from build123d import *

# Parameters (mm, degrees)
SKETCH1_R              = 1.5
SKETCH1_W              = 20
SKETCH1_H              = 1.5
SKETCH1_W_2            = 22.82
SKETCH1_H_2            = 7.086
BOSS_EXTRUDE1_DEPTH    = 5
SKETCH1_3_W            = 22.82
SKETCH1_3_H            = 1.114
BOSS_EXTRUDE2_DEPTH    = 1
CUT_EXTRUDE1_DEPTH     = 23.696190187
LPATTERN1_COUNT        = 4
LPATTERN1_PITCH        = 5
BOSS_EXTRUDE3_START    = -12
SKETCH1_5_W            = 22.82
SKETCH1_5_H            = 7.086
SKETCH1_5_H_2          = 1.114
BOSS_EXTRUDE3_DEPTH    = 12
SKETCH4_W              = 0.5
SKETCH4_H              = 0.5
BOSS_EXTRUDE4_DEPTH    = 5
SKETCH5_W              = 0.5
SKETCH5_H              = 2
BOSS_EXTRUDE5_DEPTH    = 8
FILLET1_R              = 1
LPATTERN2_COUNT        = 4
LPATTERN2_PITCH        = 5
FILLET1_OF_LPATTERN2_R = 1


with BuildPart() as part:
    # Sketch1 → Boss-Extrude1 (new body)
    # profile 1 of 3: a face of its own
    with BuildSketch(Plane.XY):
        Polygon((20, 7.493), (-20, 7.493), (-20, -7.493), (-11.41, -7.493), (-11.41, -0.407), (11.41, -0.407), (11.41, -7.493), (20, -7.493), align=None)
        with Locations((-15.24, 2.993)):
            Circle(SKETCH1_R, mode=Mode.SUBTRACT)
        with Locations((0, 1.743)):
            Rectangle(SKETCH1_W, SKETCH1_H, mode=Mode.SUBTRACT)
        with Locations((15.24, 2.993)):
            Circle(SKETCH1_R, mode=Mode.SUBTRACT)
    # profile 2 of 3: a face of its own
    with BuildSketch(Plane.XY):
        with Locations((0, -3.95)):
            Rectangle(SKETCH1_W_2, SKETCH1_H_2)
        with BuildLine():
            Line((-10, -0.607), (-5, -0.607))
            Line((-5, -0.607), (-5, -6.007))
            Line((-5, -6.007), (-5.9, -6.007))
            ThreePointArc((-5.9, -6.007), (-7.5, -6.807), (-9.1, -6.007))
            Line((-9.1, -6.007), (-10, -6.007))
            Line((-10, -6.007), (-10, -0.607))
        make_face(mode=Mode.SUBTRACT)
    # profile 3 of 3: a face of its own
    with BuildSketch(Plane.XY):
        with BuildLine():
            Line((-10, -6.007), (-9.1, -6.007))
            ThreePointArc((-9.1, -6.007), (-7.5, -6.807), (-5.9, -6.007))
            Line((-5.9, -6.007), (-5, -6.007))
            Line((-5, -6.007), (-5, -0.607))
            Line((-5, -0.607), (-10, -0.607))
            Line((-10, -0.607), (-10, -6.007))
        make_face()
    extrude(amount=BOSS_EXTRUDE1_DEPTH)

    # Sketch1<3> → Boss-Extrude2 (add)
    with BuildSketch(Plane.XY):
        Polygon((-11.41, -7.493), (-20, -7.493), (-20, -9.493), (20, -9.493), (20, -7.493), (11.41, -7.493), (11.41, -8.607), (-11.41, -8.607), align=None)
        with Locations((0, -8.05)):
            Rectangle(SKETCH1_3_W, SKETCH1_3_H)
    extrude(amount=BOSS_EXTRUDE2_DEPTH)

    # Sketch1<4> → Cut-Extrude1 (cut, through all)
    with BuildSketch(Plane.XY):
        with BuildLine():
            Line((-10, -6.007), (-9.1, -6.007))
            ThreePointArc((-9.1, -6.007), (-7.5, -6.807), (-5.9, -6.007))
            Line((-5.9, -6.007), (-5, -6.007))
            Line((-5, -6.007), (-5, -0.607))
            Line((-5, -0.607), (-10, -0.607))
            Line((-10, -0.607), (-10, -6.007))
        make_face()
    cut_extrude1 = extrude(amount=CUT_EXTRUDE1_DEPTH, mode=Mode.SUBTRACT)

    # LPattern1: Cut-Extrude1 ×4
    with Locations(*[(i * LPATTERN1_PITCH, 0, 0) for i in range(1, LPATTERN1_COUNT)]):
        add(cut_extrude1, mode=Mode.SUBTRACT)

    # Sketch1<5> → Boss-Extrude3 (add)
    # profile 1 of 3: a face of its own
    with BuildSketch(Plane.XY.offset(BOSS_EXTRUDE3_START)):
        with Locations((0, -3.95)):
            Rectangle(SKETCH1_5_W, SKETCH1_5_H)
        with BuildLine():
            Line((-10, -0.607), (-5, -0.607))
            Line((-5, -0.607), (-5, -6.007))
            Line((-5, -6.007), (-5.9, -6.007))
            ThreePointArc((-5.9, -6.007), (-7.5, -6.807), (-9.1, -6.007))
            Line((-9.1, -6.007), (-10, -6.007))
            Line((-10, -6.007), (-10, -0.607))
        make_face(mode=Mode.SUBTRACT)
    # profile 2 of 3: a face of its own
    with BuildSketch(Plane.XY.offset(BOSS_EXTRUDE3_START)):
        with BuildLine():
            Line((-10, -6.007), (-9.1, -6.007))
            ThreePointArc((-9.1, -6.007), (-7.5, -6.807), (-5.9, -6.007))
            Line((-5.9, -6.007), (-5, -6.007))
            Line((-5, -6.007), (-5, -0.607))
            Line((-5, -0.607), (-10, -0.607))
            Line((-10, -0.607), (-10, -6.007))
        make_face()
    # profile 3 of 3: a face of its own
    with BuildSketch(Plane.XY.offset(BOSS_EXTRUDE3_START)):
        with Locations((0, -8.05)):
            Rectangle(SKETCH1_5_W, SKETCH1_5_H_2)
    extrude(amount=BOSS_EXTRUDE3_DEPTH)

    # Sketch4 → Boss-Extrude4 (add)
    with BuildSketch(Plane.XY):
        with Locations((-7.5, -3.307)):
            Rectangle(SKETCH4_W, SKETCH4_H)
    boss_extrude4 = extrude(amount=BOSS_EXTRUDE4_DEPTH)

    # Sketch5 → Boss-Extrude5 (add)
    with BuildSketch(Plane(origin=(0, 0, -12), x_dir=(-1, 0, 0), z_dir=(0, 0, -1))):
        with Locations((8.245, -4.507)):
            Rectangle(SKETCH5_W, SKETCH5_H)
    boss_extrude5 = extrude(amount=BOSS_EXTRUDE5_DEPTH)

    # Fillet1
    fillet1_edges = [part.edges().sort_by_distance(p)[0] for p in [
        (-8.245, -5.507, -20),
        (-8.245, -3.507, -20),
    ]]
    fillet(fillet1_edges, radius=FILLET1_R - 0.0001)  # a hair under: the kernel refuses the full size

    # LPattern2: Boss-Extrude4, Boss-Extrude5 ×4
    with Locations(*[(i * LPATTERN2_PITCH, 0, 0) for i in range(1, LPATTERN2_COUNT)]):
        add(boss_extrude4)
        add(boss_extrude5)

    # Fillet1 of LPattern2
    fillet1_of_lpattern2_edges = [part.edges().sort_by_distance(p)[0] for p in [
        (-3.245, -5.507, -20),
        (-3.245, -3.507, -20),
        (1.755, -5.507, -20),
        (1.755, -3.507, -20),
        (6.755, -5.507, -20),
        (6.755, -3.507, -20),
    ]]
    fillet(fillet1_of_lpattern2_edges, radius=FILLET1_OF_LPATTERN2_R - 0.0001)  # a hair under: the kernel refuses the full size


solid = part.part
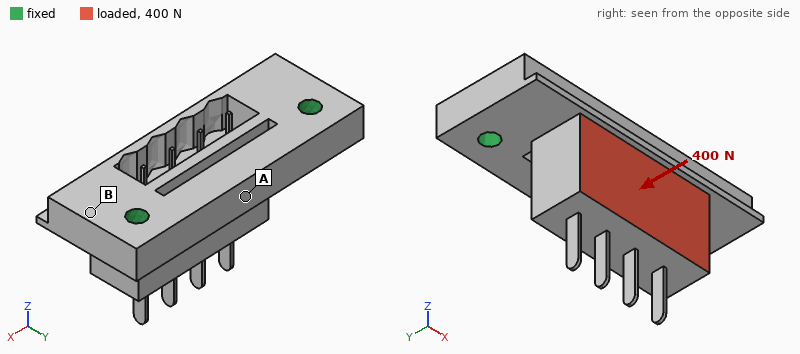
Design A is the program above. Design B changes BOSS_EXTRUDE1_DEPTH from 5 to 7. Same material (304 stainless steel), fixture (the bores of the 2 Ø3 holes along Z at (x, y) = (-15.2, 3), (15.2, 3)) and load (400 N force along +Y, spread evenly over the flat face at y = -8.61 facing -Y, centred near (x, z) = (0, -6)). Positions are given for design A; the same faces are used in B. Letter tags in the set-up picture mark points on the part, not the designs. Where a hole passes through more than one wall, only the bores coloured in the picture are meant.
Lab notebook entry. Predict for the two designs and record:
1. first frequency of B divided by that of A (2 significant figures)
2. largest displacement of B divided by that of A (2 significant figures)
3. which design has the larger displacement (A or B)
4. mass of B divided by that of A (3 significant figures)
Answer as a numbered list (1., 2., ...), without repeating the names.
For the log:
1. 1.00
2. 0.64
3. A
4. 1.19
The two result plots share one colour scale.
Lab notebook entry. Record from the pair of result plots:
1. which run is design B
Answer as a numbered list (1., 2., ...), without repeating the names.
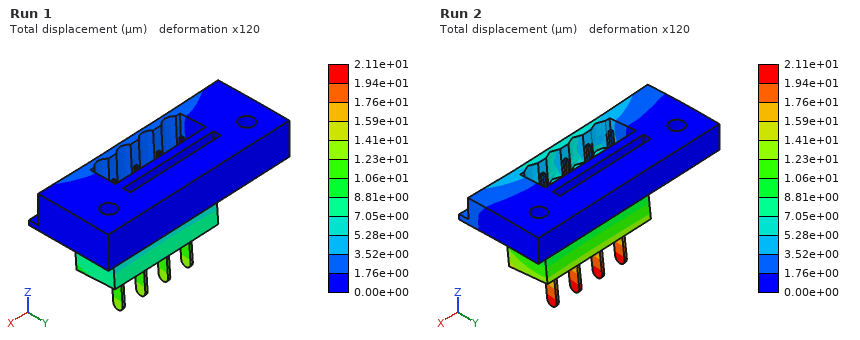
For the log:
1. Run 1
